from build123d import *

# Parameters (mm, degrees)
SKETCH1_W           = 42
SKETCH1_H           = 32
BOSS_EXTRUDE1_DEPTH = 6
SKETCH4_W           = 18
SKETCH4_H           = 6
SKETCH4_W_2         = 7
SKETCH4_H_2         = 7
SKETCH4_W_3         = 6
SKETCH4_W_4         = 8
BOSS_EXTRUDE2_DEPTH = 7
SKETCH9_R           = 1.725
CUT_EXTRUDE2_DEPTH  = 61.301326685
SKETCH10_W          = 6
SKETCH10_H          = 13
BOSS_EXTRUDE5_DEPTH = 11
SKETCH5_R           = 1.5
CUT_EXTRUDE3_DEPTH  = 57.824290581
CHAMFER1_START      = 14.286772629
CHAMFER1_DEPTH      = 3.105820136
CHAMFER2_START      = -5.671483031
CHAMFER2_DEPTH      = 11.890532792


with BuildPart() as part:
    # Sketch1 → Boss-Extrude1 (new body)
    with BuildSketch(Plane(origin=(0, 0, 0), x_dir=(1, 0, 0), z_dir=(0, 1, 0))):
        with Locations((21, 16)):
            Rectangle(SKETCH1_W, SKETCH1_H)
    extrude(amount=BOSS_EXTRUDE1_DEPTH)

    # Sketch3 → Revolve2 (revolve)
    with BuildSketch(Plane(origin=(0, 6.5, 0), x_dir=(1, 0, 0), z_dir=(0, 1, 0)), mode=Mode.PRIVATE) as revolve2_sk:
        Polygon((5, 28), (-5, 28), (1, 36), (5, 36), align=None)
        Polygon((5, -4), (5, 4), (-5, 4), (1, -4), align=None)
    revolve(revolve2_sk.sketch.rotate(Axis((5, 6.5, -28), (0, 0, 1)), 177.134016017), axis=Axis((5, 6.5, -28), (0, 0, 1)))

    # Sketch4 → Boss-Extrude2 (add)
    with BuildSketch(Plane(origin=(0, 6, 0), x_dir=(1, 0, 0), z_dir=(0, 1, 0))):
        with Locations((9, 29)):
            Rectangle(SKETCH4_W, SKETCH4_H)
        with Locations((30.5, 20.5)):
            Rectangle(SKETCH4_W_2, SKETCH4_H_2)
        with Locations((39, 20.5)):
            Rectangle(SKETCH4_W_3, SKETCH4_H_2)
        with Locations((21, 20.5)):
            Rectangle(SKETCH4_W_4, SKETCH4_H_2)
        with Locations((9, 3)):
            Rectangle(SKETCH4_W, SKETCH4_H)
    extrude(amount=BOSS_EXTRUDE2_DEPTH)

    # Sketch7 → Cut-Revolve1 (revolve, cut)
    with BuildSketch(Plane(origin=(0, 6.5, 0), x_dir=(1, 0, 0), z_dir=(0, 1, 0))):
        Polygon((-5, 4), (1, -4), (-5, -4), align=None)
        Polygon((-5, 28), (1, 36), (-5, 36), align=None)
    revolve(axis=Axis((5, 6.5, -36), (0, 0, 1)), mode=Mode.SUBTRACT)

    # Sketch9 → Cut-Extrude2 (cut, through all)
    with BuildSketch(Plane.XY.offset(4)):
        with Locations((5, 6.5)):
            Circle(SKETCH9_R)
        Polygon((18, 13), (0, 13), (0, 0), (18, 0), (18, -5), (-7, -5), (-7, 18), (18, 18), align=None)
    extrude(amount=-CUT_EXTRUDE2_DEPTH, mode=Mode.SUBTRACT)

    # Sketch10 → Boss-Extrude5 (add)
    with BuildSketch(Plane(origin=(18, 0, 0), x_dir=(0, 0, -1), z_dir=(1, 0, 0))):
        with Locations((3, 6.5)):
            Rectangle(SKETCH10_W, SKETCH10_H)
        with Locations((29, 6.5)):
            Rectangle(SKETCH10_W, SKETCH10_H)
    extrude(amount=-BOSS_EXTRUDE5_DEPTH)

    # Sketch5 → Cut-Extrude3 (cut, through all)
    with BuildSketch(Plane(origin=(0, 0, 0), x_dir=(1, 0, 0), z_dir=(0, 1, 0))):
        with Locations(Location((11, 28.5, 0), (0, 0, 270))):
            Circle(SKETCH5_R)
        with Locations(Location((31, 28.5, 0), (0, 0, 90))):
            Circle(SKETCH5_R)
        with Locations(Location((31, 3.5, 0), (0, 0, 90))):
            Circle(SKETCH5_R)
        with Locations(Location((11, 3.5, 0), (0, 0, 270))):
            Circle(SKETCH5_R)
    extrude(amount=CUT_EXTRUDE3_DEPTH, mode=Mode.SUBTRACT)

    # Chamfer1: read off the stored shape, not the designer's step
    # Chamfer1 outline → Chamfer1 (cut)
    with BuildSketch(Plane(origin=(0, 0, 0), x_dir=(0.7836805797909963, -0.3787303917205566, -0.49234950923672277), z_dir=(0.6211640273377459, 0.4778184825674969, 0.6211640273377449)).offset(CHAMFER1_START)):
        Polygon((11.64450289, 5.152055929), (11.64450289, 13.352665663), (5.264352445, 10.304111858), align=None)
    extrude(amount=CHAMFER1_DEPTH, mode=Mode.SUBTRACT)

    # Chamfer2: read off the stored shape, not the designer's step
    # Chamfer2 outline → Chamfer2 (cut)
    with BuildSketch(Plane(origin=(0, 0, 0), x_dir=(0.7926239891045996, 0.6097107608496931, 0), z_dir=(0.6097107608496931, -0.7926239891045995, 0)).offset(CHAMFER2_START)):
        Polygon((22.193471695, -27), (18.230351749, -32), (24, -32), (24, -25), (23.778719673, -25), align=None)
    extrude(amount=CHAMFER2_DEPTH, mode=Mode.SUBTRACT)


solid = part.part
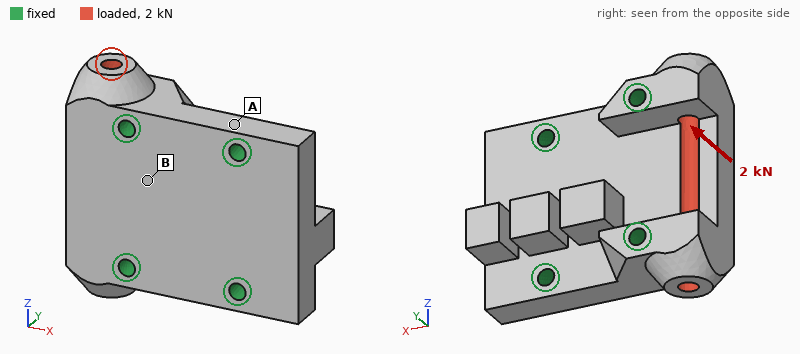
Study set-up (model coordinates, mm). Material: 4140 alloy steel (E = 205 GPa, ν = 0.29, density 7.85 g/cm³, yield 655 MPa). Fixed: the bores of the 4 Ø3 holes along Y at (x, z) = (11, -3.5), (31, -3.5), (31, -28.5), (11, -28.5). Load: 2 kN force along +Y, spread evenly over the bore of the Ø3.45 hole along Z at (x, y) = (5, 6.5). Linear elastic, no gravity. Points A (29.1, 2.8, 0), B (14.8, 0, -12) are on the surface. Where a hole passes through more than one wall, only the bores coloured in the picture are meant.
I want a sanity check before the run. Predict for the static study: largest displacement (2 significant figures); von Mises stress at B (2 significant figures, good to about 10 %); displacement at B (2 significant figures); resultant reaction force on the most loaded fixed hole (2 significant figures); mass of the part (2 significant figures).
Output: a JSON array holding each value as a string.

["2.5 µm", "8.0 MPa", "0.38 µm", "1.0 kN", "85 g"]
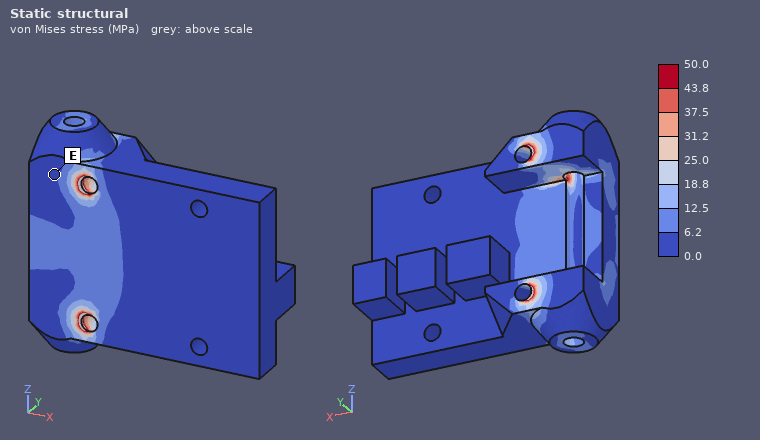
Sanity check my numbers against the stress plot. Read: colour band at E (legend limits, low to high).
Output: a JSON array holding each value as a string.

["0.0 to 6.2 MPa"]
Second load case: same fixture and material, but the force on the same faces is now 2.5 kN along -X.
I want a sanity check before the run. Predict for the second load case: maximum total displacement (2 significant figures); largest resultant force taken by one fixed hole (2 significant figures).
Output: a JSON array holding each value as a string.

["1.4 µm", "1.1 kN"]
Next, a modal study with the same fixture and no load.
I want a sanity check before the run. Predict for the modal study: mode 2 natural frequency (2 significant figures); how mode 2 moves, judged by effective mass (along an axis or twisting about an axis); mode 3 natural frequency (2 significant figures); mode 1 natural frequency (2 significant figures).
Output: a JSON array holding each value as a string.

["30 kHz", "along Y", "32 kHz", "21 kHz"]
